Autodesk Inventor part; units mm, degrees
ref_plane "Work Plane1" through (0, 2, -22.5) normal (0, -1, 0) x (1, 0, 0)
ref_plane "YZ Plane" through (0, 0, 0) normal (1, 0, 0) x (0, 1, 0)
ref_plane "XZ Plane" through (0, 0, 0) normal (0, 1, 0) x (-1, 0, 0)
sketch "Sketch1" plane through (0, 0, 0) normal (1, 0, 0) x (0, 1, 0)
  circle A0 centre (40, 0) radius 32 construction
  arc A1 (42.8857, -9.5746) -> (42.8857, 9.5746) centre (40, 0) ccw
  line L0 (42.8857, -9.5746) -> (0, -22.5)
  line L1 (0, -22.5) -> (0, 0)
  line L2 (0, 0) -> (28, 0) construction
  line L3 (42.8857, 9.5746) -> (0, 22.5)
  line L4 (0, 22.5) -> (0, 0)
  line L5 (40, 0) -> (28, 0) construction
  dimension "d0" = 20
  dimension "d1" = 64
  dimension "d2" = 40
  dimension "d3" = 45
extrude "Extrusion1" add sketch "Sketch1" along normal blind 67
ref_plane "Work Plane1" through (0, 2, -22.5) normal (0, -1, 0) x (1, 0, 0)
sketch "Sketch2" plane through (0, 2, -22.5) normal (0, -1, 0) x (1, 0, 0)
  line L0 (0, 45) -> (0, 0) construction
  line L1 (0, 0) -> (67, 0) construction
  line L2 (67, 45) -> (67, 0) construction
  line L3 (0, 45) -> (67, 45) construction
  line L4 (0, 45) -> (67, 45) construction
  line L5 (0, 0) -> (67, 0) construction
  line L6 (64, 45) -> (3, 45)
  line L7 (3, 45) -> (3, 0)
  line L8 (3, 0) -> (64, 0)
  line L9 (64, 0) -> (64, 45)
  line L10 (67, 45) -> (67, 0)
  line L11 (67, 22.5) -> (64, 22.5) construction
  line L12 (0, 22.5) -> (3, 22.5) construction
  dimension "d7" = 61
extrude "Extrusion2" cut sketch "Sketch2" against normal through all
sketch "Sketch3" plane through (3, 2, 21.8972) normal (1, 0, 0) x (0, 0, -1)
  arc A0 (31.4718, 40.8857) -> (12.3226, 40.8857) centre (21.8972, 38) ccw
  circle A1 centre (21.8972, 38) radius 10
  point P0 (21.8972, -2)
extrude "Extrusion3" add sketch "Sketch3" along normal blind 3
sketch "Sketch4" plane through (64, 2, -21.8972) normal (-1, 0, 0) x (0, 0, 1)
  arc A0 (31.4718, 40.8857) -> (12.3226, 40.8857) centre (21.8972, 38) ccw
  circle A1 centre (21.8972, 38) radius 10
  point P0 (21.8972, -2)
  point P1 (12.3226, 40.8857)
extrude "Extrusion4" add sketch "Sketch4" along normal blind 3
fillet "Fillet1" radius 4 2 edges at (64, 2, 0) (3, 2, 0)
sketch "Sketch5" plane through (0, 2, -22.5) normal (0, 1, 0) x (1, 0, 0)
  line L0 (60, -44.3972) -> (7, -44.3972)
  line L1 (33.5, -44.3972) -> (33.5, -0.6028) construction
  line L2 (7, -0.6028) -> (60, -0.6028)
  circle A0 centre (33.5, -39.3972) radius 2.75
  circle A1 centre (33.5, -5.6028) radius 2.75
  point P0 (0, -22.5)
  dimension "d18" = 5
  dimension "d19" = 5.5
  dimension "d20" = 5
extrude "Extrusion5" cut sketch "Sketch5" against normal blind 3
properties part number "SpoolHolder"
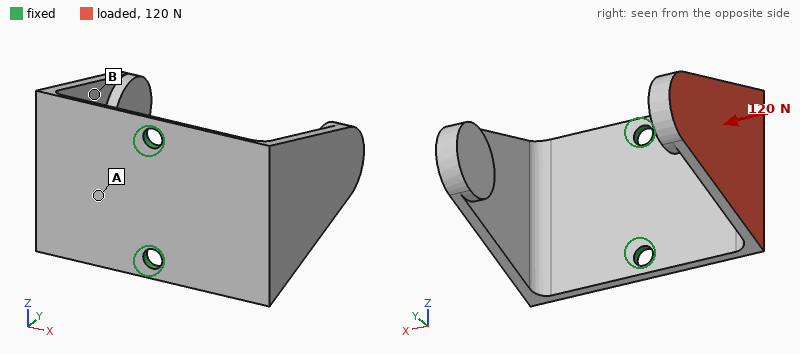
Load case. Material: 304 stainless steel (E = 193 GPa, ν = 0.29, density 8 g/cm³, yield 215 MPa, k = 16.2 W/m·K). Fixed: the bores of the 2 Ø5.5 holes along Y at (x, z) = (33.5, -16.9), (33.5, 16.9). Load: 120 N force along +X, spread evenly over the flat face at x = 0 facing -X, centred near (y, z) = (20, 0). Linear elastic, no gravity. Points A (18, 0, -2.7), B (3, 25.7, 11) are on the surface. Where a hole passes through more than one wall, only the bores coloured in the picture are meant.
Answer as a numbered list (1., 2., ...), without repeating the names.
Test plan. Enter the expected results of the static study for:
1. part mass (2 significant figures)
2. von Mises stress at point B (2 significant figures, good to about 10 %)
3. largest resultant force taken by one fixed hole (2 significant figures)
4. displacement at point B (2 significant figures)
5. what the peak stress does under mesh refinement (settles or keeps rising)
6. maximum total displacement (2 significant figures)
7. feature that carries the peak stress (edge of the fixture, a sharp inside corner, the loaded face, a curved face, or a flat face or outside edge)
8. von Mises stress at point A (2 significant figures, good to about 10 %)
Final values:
1. 130 g
2. 11 MPa
3. 62 N
4. 0.34 mm
5. keeps rising
6. 0.63 mm
7. edge of the fixture
8. 68 MPa
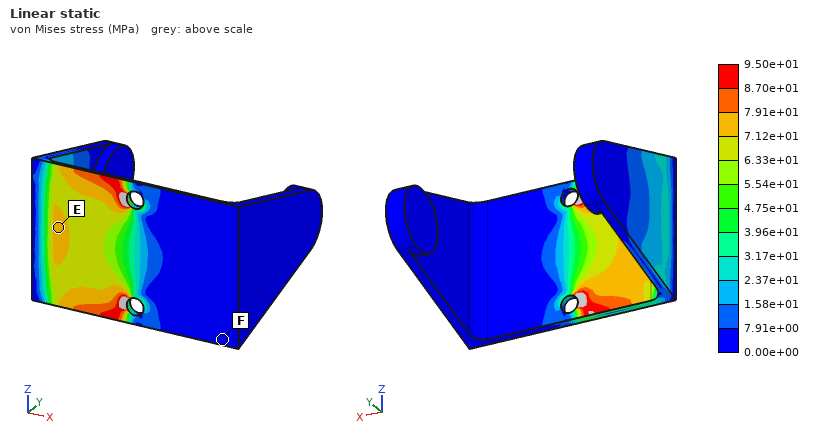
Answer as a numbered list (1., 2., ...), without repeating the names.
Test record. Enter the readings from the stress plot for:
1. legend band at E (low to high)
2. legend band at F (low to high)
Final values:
1. 7.12e+01 to 7.91e+01 MPa
2. 0.00e+00 to 7.91e+00 MPa
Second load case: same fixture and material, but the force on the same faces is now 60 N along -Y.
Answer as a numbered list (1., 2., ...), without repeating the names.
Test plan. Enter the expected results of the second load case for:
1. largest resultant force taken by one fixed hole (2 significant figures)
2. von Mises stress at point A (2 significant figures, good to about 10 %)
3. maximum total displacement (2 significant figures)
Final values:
1. 30 N
2. 33 MPa
3. 0.29 mm
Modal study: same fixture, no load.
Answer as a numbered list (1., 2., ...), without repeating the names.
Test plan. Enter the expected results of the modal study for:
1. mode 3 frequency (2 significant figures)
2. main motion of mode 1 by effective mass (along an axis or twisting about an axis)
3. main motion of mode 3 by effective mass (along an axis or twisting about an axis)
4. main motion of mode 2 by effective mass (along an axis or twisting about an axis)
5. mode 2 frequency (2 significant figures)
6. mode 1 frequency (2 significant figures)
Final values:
1. 730 Hz
2. along X
3. twisting about Y
4. along Y
5. 340 Hz
6. 320 Hz
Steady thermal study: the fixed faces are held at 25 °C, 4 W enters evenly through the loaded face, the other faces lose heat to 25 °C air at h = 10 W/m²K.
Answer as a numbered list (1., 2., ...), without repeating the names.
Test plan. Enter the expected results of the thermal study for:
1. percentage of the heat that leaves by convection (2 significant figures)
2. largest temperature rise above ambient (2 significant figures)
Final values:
1. 53 %
2. 74 K
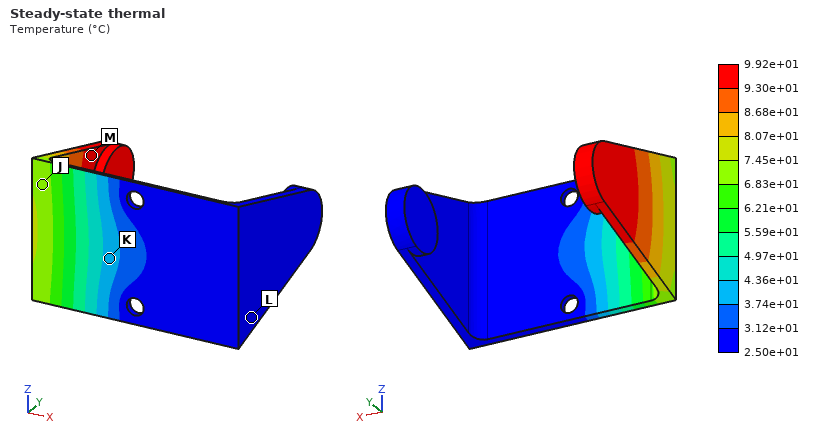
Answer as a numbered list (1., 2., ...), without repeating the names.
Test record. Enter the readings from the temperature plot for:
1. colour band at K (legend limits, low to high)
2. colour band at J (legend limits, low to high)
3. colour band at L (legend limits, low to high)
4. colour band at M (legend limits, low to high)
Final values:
1. 3.74e+01 to 4.36e+01 °C
2. 6.83e+01 to 7.45e+01 °C
3. 2.50e+01 to 3.12e+01 °C
4. 9.30e+01 to 9.92e+01 °C
